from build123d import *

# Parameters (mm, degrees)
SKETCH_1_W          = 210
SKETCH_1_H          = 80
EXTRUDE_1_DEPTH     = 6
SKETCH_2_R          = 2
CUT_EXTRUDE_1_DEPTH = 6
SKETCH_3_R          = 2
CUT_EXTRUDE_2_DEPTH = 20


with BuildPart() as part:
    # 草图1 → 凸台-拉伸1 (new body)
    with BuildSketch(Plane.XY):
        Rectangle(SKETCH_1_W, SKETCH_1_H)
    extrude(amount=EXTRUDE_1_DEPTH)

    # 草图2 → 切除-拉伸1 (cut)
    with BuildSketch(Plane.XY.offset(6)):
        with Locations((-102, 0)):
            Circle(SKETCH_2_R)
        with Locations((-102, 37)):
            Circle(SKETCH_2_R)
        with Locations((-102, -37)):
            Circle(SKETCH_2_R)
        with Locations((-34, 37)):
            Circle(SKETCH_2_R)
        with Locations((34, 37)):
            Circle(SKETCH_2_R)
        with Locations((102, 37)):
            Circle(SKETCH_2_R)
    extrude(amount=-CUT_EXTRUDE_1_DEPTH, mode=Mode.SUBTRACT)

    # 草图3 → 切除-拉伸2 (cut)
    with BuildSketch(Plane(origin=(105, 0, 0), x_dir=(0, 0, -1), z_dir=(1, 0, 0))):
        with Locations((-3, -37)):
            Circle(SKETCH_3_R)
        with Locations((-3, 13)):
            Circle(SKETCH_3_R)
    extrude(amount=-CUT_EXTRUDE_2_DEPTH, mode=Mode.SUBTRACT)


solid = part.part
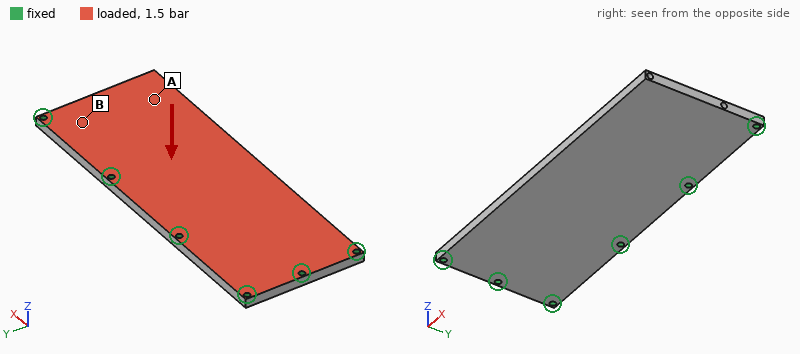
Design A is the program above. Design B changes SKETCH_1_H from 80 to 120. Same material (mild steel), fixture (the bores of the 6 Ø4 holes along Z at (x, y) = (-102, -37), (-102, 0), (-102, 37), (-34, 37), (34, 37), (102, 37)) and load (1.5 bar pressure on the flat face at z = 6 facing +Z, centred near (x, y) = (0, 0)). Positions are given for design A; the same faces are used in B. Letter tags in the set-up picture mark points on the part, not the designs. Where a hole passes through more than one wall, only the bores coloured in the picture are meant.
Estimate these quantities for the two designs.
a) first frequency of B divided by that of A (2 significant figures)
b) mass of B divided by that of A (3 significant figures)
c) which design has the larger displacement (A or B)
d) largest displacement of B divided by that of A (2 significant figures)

0.76
1.50
B
1.8
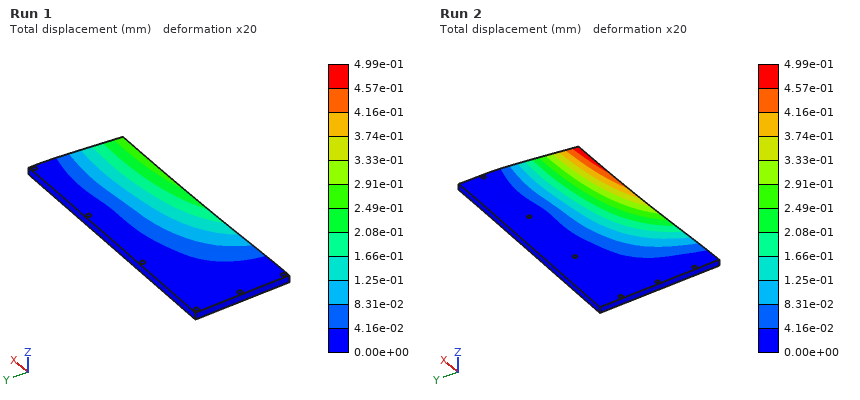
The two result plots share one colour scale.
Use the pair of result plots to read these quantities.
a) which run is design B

Run 2
